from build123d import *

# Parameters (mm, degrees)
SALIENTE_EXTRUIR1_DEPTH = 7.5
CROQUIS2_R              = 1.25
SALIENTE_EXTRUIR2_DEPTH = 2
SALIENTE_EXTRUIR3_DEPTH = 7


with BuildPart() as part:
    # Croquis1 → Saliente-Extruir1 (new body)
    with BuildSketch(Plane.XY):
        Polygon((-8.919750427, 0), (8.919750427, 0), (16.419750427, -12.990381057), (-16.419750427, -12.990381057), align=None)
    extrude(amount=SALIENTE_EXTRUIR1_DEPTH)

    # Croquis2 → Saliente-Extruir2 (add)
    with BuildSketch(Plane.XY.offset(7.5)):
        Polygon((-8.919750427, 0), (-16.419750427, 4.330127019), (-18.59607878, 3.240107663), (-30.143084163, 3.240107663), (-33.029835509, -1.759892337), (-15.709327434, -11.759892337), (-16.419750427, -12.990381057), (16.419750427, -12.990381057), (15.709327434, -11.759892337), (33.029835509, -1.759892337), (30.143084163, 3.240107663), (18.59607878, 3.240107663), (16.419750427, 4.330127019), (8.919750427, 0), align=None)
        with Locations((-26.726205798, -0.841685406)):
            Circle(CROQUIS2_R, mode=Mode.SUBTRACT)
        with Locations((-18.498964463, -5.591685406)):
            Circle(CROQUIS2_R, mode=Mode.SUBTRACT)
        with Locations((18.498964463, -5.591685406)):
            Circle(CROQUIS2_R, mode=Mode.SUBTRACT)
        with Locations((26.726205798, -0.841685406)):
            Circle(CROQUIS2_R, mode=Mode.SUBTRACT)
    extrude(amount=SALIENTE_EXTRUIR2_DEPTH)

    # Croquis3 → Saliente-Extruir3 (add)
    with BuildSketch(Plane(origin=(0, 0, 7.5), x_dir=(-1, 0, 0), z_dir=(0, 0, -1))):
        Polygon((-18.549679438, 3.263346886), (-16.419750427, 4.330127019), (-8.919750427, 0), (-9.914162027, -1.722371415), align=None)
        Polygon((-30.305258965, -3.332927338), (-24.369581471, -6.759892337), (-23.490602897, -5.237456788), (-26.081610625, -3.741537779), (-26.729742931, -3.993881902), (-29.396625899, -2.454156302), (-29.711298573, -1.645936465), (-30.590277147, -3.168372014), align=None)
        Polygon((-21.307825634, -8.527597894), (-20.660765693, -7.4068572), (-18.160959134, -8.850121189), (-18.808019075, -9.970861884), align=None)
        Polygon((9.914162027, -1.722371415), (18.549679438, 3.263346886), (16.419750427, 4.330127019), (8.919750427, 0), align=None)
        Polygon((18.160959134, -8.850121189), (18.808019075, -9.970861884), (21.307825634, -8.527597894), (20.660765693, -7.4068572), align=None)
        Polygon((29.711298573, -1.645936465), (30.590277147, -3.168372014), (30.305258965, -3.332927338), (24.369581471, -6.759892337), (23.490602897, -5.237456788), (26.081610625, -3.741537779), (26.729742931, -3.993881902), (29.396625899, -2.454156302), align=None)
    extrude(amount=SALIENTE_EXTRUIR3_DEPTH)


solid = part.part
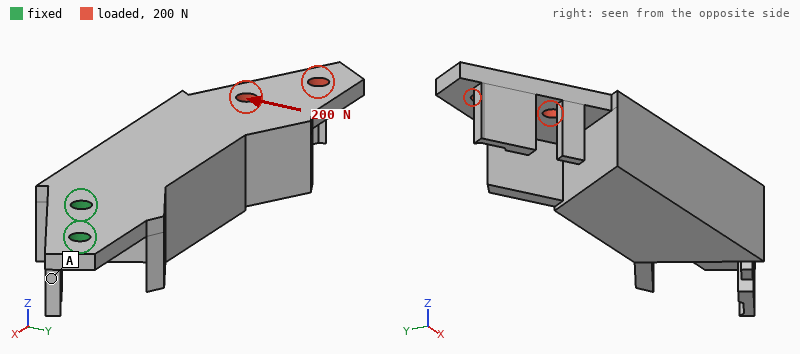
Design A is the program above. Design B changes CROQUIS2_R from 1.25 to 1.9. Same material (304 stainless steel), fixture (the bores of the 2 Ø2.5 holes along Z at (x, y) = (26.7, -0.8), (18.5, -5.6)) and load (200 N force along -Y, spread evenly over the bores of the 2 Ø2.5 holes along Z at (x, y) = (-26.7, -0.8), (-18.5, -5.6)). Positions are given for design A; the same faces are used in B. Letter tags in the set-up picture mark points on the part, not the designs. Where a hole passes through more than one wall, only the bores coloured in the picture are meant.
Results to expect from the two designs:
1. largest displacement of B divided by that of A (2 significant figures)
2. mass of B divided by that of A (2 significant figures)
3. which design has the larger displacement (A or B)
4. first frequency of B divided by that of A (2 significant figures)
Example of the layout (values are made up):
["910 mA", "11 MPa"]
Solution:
["0.87", "0.99", "A", "1.1"]
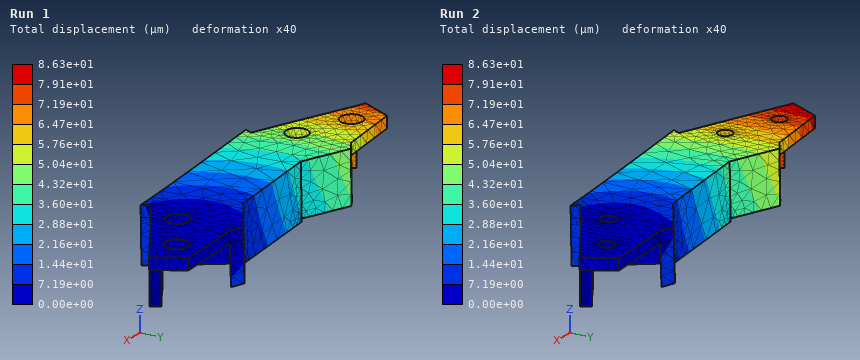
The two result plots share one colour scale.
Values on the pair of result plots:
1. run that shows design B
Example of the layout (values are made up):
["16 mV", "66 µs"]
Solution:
["Run 1"]
